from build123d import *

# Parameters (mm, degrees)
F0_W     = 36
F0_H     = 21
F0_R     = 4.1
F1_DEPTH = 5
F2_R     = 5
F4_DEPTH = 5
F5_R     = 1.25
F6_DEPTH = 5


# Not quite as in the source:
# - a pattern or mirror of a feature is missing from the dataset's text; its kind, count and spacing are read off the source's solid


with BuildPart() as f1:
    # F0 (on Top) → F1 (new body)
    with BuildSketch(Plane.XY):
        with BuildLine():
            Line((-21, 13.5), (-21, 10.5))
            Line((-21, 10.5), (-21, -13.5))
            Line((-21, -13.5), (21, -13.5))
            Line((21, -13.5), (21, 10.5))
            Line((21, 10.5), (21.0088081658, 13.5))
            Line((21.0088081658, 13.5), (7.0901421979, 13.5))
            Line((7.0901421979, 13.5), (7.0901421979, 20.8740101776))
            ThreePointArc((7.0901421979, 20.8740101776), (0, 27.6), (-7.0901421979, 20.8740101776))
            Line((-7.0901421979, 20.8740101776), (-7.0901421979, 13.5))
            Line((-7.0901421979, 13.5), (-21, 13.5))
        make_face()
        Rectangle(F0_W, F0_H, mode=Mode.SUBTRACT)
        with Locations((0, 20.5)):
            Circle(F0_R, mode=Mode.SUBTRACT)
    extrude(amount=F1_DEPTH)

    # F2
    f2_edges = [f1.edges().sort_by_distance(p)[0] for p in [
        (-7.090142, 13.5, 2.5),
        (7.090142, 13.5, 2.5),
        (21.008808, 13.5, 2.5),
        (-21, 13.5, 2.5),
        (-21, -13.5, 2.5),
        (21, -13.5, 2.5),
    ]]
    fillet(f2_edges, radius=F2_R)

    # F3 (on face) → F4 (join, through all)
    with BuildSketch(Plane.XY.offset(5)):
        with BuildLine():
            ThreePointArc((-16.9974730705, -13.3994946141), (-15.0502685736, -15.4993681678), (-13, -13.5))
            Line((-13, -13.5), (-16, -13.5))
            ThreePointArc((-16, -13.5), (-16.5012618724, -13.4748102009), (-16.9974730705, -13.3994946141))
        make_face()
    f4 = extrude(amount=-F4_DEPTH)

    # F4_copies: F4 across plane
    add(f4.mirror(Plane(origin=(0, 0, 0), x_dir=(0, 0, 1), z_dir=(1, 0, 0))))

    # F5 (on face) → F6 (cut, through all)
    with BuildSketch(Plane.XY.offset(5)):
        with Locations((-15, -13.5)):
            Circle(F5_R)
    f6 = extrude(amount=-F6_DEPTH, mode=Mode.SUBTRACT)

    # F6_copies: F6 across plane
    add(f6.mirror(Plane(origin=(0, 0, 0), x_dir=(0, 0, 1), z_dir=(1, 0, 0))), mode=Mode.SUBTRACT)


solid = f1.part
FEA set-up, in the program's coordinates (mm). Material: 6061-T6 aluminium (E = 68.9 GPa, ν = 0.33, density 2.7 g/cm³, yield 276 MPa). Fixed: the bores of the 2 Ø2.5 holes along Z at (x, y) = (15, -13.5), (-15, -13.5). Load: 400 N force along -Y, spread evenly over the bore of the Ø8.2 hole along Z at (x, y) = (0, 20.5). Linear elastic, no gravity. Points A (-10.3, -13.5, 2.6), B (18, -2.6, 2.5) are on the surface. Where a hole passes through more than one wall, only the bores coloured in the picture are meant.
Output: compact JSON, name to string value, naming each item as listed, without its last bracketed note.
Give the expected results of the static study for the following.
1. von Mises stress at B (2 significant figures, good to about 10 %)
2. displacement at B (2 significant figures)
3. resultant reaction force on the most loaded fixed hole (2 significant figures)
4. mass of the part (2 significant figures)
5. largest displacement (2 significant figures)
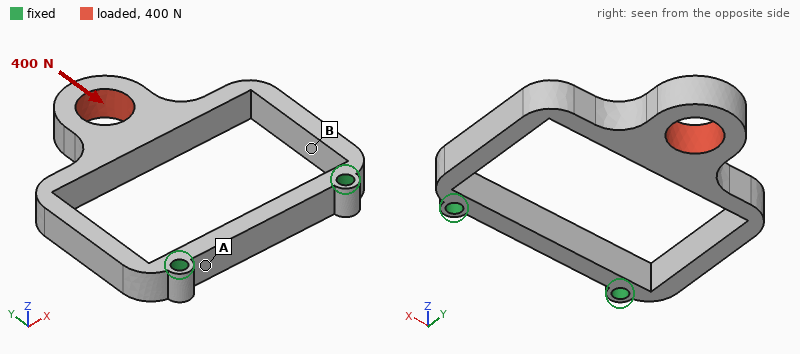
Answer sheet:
{"von Mises stress at B": "45 MPa", "displacement at B": "29 µm", "resultant reaction force on the most loaded fixed hole": "200 N", "mass of the part": "6.7 g", "largest displacement": "98 µm"}
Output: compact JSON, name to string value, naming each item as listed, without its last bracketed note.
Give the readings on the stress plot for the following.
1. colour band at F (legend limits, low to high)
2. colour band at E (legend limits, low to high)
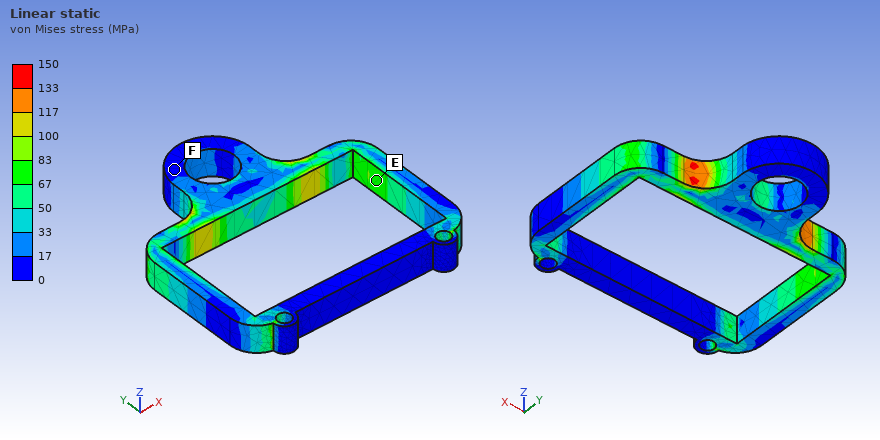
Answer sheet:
{"colour band at F": "0 to 17 MPa", "colour band at E": "67 to 83 MPa"}
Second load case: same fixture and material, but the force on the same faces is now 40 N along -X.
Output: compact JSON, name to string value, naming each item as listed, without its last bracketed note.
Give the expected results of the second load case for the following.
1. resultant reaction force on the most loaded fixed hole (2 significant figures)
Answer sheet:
{"resultant reaction force on the most loaded fixed hole": "30 N"}
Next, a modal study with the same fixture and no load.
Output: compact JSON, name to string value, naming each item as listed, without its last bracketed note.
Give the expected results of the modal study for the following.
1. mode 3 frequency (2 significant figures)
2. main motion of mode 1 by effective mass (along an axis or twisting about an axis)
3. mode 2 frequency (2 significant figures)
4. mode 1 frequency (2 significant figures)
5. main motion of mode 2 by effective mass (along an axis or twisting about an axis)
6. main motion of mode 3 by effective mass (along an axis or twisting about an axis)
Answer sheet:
{"mode 3 frequency": "4600 Hz", "main motion of mode 1 by effective mass": "along Z", "mode 2 frequency": "1800 Hz", "mode 1 frequency": "1400 Hz", "main motion of mode 2 by effective mass": "along X", "main motion of mode 3 by effective mass": "twisting about Y"}
